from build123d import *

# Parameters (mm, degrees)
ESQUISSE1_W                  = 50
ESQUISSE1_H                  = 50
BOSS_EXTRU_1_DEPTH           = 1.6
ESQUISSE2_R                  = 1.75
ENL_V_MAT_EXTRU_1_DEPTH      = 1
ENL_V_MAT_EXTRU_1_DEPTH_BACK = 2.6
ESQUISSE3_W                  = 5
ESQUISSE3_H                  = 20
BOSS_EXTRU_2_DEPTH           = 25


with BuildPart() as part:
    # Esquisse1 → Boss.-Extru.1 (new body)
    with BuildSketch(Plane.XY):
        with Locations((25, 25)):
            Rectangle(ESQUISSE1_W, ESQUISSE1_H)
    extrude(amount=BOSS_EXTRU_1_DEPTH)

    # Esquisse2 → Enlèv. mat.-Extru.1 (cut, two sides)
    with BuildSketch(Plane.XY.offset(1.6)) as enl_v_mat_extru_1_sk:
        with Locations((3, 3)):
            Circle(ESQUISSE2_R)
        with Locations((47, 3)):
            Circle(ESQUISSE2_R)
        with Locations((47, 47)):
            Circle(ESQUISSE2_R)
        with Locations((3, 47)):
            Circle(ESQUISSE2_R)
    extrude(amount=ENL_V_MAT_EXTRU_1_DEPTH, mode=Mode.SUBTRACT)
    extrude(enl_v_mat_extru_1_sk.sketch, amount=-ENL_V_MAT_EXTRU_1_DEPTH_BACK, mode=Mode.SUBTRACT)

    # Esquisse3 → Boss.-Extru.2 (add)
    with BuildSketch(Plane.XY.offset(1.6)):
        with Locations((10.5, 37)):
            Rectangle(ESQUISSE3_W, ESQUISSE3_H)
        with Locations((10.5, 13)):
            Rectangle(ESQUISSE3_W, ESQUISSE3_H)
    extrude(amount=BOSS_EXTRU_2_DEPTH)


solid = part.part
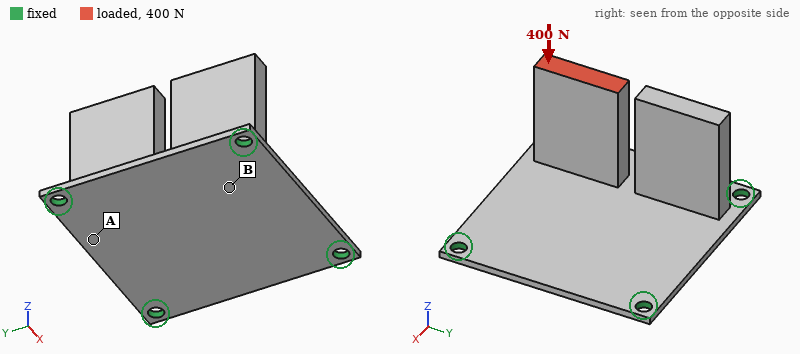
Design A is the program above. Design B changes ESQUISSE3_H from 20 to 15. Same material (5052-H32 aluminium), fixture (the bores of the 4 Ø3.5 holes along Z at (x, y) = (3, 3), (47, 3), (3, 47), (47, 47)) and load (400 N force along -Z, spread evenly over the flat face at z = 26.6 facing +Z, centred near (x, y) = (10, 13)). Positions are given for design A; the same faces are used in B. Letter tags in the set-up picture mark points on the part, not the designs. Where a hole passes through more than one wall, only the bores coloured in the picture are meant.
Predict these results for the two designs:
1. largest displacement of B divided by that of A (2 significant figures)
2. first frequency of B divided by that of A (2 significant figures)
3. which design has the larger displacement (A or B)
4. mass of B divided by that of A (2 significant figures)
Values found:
1.2
1.1
B
0.86
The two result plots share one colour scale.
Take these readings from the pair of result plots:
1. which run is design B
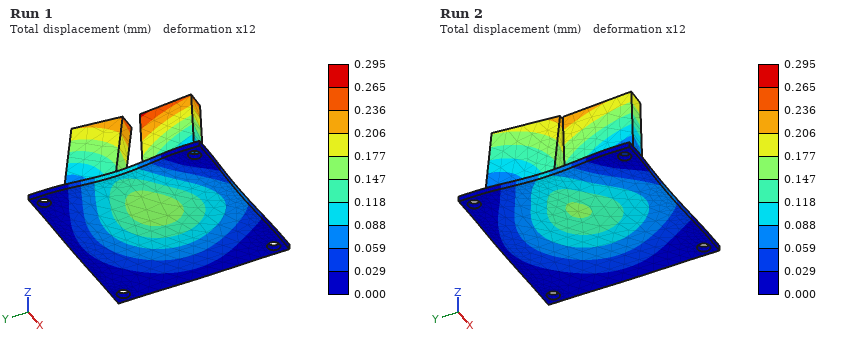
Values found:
Run 1
